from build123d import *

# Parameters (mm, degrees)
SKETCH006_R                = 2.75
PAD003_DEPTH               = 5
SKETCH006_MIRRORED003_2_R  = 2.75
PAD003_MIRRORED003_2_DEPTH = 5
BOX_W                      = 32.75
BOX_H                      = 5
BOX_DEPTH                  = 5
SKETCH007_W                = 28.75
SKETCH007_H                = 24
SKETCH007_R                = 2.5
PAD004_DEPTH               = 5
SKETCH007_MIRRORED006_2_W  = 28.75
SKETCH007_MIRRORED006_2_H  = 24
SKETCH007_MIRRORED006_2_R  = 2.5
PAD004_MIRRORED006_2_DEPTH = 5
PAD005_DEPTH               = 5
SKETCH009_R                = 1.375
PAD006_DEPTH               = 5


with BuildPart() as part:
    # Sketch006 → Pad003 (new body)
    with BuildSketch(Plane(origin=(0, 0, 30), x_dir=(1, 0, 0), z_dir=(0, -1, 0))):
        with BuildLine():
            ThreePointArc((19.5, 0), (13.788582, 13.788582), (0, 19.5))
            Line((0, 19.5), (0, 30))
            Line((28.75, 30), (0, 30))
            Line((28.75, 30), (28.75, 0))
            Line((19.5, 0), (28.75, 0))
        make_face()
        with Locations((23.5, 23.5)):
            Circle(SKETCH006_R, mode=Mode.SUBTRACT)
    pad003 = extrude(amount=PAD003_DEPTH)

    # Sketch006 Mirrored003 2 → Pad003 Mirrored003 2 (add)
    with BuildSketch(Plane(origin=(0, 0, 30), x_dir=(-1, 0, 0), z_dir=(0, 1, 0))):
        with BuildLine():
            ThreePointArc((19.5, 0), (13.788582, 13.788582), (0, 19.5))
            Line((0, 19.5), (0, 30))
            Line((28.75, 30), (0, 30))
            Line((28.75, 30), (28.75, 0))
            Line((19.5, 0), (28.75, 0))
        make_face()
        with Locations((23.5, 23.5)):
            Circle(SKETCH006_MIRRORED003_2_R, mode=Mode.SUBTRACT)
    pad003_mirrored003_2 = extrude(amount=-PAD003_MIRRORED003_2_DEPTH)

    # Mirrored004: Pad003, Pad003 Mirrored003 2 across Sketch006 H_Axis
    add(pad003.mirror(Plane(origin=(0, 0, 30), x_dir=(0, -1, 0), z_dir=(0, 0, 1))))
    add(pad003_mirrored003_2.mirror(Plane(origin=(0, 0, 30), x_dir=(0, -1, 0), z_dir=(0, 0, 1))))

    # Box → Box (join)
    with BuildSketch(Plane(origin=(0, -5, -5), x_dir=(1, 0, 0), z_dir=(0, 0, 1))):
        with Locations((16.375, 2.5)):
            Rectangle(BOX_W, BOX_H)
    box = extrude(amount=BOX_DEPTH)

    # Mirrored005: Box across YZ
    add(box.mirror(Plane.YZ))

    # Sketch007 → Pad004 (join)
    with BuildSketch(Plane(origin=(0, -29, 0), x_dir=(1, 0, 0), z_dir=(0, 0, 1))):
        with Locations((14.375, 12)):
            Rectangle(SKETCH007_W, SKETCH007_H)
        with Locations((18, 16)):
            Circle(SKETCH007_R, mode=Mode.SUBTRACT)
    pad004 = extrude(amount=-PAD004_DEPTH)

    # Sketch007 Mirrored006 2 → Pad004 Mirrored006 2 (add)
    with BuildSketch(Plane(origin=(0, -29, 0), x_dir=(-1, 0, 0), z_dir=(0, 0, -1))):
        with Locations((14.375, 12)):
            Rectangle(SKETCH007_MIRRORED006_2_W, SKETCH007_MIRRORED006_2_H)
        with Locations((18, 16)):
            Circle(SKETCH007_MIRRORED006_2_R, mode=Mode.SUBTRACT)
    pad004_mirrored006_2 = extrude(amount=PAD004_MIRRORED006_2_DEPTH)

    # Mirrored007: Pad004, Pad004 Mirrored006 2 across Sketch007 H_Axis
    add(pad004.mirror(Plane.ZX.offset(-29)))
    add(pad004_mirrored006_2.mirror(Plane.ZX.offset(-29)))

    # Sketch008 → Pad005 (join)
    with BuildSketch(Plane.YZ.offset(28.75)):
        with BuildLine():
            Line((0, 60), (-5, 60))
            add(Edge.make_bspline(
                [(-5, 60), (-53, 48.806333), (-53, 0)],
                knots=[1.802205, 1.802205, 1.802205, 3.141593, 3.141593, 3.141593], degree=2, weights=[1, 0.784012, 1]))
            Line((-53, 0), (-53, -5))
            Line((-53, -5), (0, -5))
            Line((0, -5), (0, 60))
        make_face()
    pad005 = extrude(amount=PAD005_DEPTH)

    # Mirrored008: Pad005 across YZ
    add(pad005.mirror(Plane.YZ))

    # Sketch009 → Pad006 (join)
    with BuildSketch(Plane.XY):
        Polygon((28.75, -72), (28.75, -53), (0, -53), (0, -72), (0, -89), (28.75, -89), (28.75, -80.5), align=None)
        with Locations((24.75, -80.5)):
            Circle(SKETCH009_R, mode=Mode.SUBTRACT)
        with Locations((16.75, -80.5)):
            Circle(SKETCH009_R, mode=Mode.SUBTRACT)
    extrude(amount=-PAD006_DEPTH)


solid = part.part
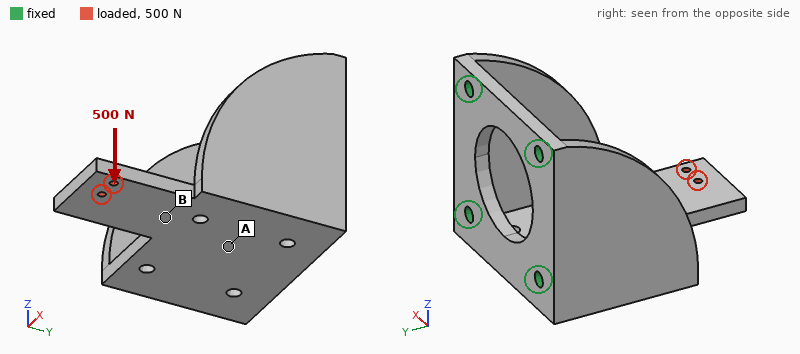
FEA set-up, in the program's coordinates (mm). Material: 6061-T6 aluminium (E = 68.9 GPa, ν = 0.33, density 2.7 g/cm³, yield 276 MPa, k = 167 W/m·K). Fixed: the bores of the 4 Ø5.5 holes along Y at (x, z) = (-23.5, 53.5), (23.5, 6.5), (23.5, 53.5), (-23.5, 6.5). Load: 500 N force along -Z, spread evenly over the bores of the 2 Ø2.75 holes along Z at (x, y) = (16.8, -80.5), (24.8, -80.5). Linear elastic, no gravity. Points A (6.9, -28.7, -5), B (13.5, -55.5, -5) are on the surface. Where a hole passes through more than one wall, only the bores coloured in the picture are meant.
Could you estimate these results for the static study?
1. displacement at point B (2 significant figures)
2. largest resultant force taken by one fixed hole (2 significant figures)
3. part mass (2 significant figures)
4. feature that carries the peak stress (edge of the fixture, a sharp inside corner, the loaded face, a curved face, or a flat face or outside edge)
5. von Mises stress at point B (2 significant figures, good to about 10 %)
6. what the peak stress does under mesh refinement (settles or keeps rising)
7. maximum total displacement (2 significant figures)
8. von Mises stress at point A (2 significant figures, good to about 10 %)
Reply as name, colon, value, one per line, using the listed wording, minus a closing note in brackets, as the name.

displacement at point B: 0.14 mm
largest resultant force taken by one fixed hole: 720 N
part mass: 160 g
feature that carries the peak stress: a sharp inside corner
von Mises stress at point B: 95 MPa
what the peak stress does under mesh refinement: keeps rising
maximum total displacement: 0.65 mm
von Mises stress at point A: 18 MPa
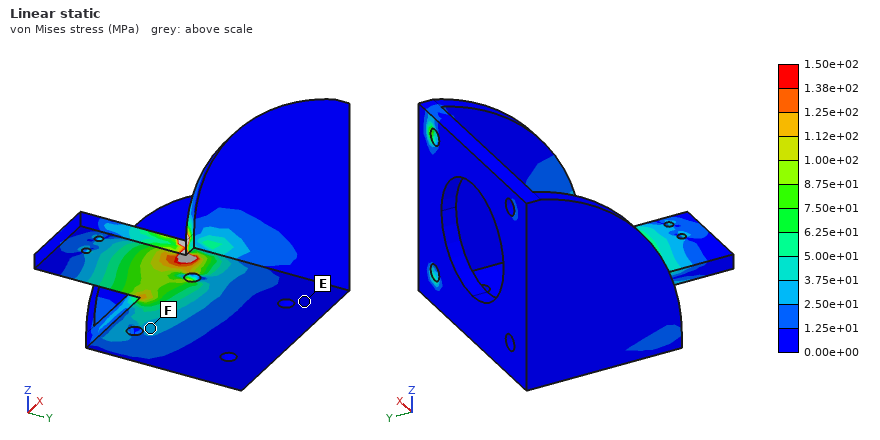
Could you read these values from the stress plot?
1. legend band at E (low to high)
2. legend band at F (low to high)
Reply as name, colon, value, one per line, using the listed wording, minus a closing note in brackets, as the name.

legend band at E: 0.00e+00 to 1.25e+01 MPa
legend band at F: 2.50e+01 to 3.75e+01 MPa
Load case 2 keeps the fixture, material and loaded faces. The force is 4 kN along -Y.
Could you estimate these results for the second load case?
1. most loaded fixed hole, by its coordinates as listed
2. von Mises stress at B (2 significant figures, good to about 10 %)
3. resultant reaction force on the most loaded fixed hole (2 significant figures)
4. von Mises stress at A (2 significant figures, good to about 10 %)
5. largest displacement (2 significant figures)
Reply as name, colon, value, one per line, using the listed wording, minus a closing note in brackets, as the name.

most loaded fixed hole, by its coordinates as listed: (23.5, 6.5)
von Mises stress at B: 25 MPa
resultant reaction force on the most loaded fixed hole: 4.0 kN
von Mises stress at A: 15 MPa
largest displacement: 0.13 mm
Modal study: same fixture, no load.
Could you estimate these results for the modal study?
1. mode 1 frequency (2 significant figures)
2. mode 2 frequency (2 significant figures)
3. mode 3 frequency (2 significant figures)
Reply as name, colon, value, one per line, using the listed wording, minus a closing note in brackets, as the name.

mode 1 frequency: 1700 Hz
mode 2 frequency: 3600 Hz
mode 3 frequency: 3600 Hz
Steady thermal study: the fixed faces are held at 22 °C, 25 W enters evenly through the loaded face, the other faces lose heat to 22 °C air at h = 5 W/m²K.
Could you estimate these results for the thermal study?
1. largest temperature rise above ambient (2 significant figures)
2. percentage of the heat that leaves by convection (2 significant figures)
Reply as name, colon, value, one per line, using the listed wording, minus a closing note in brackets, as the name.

largest temperature rise above ambient: 60 K
percentage of the heat that leaves by convection: 4.6 %
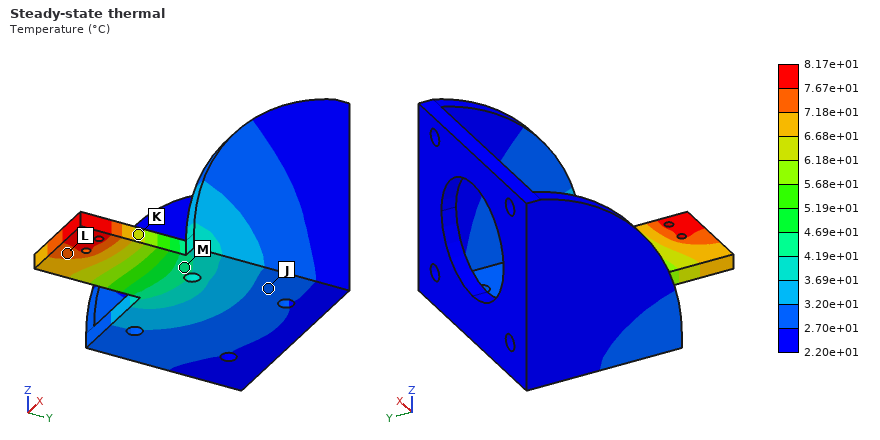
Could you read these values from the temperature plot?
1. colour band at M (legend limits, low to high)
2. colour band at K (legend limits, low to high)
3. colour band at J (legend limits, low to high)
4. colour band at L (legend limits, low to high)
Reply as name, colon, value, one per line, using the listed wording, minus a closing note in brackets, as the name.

colour band at M: 4.19e+01 to 4.69e+01 °C
colour band at K: 6.18e+01 to 6.68e+01 °C
colour band at J: 2.70e+01 to 3.20e+01 °C
colour band at L: 7.18e+01 to 7.67e+01 °C
